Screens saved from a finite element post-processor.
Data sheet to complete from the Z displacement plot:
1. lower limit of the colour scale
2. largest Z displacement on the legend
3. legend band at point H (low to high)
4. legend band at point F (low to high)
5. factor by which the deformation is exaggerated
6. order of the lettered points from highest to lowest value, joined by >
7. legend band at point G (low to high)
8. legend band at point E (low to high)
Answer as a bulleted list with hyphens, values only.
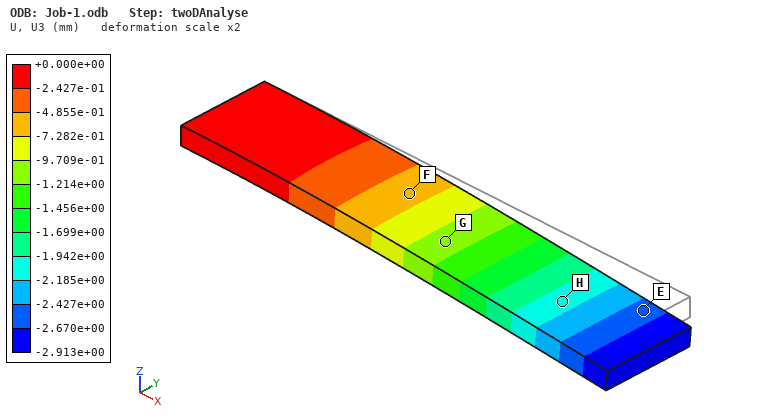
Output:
- -2.913e+00 mm
- +0.000e+00 mm
- -2.185e+00 to -1.942e+00 mm
- -7.282e-01 to -4.855e-01 mm
- 2
- F > G > H > E
- -1.214e+00 to -9.709e-01 mm
- -2.670e+00 to -2.427e+00 mm
